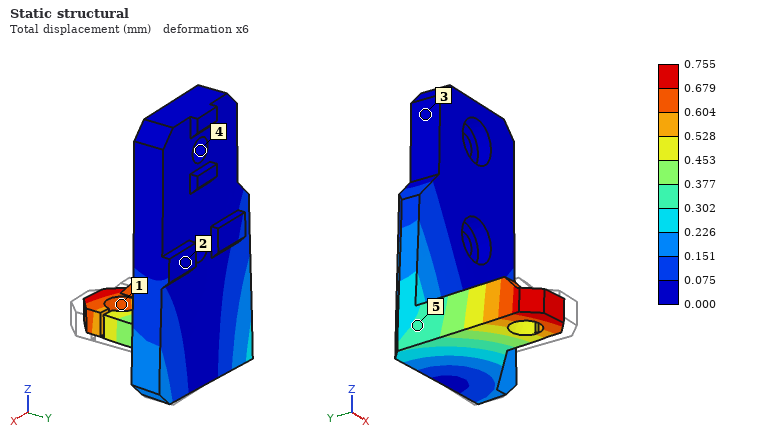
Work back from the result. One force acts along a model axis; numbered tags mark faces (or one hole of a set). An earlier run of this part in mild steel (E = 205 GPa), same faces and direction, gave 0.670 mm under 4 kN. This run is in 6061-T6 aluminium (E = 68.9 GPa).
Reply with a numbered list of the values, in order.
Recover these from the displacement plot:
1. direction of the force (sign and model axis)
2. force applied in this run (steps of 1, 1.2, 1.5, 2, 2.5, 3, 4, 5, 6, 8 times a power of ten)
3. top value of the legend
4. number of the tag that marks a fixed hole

1. -X
2. 1.5 kN
3. 0.755 mm
4. 4
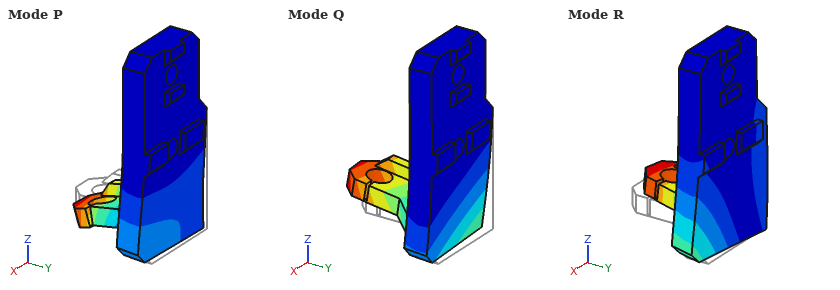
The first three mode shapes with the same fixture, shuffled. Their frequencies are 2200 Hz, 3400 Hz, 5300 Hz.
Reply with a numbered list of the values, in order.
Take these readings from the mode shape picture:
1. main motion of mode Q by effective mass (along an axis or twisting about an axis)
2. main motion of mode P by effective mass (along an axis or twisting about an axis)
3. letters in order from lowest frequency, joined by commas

1. along Y
2. along Y
3. Q, R, P
